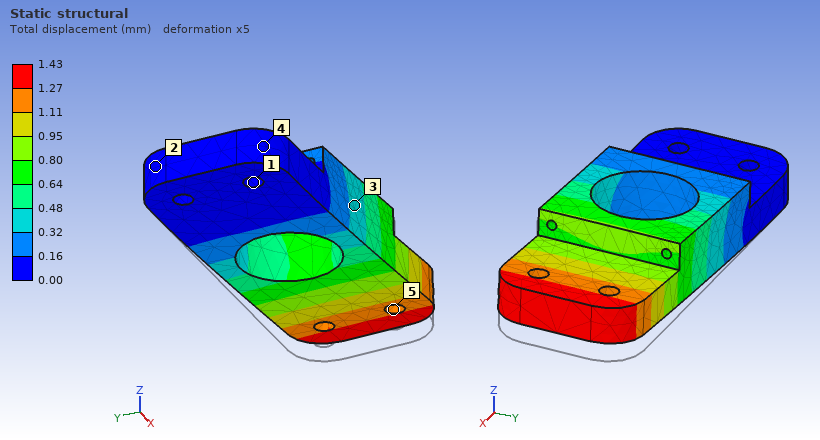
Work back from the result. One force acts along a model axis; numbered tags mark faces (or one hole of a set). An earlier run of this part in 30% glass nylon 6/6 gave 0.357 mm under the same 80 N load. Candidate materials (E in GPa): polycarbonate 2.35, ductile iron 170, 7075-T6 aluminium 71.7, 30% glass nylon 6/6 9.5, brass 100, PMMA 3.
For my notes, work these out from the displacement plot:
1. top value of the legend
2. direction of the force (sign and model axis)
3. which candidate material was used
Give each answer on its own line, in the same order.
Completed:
1.43 mm
+Z
polycarbonate
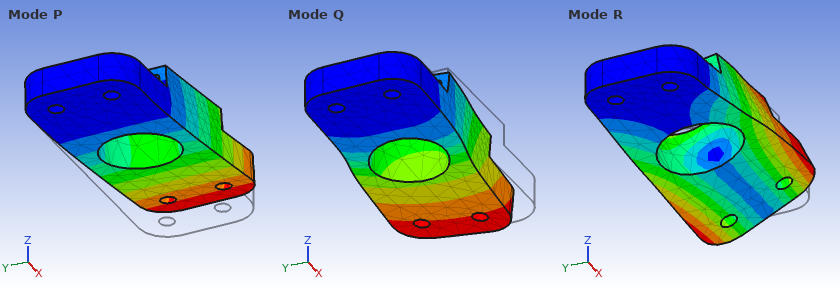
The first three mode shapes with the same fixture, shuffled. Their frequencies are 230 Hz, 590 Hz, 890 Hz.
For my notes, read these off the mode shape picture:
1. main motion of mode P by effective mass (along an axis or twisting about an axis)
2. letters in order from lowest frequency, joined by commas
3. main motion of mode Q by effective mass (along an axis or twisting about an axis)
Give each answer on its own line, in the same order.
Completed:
along Z
P, Q, R
along Y
